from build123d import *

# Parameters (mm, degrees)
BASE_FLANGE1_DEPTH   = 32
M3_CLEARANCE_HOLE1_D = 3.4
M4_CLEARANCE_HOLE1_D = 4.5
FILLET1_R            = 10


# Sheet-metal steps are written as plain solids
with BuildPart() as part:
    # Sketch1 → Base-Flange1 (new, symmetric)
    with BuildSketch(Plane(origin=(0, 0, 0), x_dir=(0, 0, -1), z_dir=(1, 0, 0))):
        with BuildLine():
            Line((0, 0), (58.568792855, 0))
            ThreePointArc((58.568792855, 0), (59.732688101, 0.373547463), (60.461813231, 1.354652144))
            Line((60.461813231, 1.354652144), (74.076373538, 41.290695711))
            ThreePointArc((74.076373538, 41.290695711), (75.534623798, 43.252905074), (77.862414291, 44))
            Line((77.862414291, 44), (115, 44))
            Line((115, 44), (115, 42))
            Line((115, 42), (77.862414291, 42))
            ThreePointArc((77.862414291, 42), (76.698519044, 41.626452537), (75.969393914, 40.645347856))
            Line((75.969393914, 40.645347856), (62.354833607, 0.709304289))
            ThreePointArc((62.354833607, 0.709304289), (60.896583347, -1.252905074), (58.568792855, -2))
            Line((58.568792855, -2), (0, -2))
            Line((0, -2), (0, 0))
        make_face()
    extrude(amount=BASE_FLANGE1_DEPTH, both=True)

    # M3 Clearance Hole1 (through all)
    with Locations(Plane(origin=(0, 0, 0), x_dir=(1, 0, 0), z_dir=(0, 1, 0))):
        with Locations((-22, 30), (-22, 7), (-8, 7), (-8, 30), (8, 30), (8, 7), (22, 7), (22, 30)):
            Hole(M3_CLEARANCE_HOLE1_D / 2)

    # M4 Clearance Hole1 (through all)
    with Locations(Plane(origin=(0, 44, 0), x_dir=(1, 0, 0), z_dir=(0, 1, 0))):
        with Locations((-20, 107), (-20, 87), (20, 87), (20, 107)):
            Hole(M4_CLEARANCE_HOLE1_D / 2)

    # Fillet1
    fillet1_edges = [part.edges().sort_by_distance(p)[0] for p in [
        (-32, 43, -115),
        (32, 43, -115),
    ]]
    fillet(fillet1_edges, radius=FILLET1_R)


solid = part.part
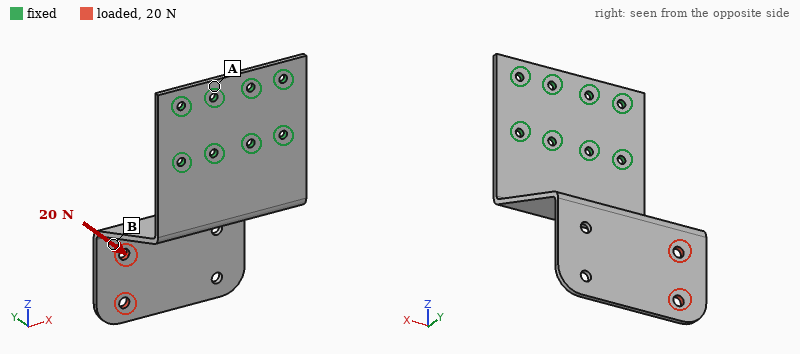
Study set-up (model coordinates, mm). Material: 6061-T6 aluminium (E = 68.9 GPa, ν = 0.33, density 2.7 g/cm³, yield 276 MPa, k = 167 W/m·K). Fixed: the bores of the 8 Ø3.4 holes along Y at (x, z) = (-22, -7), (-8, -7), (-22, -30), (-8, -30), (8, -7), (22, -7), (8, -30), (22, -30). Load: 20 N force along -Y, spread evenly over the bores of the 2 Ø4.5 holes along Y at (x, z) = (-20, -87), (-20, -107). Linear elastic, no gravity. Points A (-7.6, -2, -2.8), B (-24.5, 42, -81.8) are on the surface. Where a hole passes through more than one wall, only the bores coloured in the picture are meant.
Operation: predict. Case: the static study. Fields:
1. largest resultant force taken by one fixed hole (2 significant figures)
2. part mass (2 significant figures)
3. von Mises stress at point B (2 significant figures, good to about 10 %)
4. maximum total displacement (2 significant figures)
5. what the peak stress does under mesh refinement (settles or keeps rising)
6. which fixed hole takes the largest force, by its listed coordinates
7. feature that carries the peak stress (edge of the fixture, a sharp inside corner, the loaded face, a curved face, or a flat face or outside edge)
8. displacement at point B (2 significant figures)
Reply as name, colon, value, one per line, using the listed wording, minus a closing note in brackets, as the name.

largest resultant force taken by one fixed hole: 14 N
part mass: 49 g
von Mises stress at point B: 7.9 MPa
maximum total displacement: 1.4 mm
what the peak stress does under mesh refinement: keeps rising
which fixed hole takes the largest force, by its listed coordinates: (-22, -30)
feature that carries the peak stress: edge of the fixture
displacement at point B: 0.85 mm
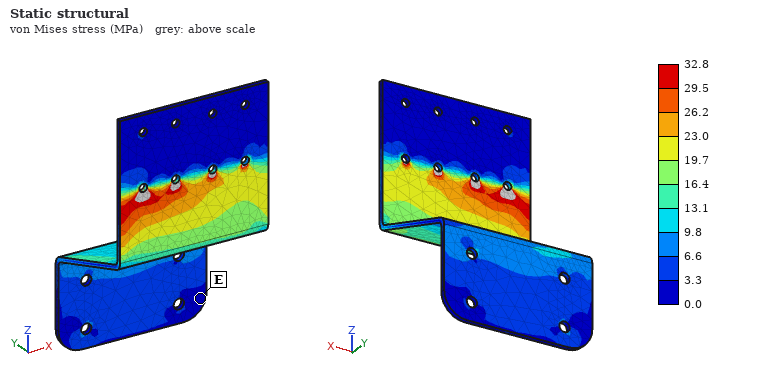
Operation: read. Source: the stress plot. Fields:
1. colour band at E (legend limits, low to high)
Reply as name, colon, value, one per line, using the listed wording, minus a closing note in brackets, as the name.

colour band at E: 0.0 to 3.3 MPa
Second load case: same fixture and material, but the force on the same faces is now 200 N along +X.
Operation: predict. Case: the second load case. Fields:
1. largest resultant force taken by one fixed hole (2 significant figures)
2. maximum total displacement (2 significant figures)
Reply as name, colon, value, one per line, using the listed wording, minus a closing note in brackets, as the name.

largest resultant force taken by one fixed hole: 290 N
maximum total displacement: 1.5 mm
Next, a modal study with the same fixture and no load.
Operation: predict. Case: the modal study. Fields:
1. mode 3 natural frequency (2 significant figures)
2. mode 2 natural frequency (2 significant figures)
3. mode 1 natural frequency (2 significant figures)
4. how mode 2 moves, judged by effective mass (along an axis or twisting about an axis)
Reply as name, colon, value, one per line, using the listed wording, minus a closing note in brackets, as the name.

mode 3 natural frequency: 550 Hz
mode 2 natural frequency: 470 Hz
mode 1 natural frequency: 160 Hz
how mode 2 moves, judged by effective mass: along X
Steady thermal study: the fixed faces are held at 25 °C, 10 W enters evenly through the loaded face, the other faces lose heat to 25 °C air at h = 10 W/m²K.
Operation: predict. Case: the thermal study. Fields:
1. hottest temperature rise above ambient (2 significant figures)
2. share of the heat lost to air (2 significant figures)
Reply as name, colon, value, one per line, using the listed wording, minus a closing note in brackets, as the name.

hottest temperature rise above ambient: 45 K
share of the heat lost to air: 30 %
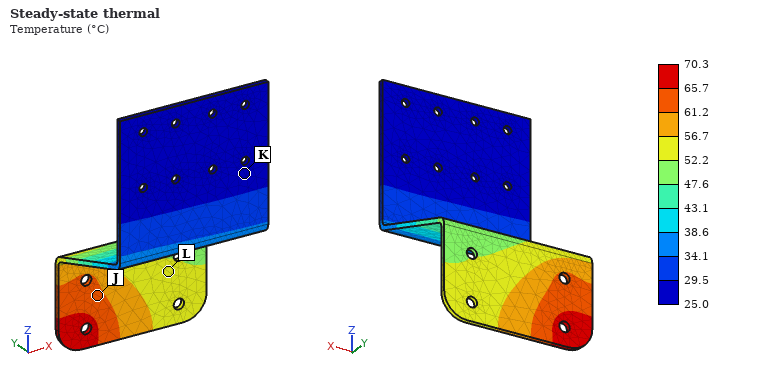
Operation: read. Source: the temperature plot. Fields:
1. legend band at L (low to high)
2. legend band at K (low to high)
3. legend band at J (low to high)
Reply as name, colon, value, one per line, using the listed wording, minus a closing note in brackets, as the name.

legend band at L: 52.2 to 56.7 °C
legend band at K: 25.0 to 29.5 °C
legend band at J: 61.2 to 65.7 °C
